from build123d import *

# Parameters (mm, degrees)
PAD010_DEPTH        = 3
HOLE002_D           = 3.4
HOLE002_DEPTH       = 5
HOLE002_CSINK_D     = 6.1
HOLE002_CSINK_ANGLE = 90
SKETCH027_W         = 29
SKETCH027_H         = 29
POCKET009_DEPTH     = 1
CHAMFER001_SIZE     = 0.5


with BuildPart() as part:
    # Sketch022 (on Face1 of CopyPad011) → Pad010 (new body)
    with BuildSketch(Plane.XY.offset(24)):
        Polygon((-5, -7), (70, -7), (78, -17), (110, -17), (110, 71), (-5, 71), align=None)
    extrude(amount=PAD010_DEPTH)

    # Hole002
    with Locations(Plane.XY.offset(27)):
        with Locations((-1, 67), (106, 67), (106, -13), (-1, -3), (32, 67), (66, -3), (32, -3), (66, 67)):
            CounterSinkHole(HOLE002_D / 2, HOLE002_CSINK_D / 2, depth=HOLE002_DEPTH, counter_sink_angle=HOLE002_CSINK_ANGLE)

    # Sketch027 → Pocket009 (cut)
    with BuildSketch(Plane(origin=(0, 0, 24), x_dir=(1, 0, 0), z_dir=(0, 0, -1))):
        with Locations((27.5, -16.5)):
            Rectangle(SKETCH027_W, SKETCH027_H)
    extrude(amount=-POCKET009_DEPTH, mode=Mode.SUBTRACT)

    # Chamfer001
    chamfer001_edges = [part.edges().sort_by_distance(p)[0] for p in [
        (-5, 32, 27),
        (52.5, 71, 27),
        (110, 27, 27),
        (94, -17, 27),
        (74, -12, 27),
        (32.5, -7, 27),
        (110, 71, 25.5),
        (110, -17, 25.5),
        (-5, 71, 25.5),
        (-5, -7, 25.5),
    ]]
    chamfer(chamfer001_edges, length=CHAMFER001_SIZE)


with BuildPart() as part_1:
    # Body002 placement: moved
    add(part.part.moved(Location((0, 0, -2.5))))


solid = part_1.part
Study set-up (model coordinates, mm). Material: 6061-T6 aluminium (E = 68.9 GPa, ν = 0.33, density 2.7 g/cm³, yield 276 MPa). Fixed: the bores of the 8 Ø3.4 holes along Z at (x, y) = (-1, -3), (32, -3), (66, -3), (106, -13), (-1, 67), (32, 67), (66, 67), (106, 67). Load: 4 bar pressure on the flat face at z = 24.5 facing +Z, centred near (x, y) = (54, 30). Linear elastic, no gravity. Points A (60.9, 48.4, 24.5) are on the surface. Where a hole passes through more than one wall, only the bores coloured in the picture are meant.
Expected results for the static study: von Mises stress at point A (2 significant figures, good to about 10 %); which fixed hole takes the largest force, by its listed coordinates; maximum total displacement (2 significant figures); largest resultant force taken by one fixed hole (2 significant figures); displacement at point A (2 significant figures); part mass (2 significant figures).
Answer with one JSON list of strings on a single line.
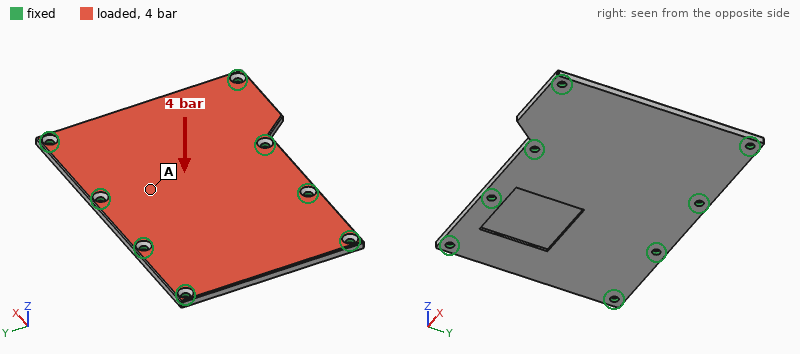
["44 MPa", "(66, -3)", "0.39 mm", "940 N", "0.19 mm", "72 g"]
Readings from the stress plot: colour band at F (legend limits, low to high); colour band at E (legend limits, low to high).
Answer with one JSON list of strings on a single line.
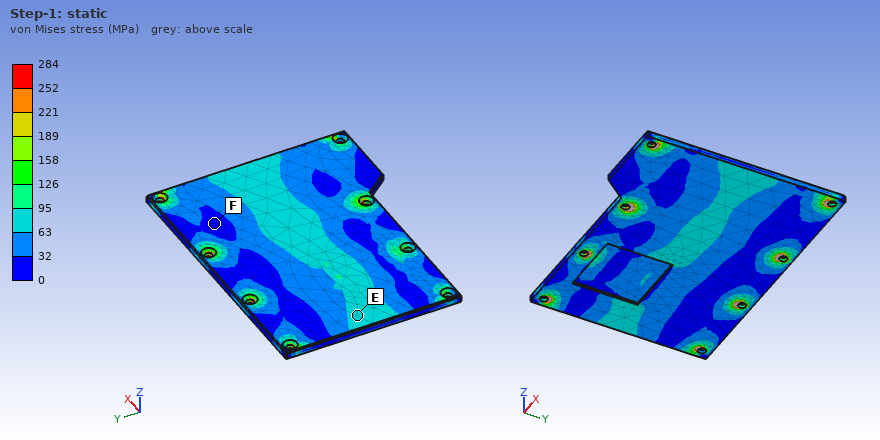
["0 to 32 MPa", "63 to 95 MPa"]
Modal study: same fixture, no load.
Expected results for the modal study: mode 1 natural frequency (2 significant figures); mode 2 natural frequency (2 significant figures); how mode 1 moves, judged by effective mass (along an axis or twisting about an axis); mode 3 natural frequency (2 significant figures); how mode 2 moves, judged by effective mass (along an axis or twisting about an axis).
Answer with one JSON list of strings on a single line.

["2200 Hz", "2700 Hz", "along Z", "3600 Hz", "along Z"]
